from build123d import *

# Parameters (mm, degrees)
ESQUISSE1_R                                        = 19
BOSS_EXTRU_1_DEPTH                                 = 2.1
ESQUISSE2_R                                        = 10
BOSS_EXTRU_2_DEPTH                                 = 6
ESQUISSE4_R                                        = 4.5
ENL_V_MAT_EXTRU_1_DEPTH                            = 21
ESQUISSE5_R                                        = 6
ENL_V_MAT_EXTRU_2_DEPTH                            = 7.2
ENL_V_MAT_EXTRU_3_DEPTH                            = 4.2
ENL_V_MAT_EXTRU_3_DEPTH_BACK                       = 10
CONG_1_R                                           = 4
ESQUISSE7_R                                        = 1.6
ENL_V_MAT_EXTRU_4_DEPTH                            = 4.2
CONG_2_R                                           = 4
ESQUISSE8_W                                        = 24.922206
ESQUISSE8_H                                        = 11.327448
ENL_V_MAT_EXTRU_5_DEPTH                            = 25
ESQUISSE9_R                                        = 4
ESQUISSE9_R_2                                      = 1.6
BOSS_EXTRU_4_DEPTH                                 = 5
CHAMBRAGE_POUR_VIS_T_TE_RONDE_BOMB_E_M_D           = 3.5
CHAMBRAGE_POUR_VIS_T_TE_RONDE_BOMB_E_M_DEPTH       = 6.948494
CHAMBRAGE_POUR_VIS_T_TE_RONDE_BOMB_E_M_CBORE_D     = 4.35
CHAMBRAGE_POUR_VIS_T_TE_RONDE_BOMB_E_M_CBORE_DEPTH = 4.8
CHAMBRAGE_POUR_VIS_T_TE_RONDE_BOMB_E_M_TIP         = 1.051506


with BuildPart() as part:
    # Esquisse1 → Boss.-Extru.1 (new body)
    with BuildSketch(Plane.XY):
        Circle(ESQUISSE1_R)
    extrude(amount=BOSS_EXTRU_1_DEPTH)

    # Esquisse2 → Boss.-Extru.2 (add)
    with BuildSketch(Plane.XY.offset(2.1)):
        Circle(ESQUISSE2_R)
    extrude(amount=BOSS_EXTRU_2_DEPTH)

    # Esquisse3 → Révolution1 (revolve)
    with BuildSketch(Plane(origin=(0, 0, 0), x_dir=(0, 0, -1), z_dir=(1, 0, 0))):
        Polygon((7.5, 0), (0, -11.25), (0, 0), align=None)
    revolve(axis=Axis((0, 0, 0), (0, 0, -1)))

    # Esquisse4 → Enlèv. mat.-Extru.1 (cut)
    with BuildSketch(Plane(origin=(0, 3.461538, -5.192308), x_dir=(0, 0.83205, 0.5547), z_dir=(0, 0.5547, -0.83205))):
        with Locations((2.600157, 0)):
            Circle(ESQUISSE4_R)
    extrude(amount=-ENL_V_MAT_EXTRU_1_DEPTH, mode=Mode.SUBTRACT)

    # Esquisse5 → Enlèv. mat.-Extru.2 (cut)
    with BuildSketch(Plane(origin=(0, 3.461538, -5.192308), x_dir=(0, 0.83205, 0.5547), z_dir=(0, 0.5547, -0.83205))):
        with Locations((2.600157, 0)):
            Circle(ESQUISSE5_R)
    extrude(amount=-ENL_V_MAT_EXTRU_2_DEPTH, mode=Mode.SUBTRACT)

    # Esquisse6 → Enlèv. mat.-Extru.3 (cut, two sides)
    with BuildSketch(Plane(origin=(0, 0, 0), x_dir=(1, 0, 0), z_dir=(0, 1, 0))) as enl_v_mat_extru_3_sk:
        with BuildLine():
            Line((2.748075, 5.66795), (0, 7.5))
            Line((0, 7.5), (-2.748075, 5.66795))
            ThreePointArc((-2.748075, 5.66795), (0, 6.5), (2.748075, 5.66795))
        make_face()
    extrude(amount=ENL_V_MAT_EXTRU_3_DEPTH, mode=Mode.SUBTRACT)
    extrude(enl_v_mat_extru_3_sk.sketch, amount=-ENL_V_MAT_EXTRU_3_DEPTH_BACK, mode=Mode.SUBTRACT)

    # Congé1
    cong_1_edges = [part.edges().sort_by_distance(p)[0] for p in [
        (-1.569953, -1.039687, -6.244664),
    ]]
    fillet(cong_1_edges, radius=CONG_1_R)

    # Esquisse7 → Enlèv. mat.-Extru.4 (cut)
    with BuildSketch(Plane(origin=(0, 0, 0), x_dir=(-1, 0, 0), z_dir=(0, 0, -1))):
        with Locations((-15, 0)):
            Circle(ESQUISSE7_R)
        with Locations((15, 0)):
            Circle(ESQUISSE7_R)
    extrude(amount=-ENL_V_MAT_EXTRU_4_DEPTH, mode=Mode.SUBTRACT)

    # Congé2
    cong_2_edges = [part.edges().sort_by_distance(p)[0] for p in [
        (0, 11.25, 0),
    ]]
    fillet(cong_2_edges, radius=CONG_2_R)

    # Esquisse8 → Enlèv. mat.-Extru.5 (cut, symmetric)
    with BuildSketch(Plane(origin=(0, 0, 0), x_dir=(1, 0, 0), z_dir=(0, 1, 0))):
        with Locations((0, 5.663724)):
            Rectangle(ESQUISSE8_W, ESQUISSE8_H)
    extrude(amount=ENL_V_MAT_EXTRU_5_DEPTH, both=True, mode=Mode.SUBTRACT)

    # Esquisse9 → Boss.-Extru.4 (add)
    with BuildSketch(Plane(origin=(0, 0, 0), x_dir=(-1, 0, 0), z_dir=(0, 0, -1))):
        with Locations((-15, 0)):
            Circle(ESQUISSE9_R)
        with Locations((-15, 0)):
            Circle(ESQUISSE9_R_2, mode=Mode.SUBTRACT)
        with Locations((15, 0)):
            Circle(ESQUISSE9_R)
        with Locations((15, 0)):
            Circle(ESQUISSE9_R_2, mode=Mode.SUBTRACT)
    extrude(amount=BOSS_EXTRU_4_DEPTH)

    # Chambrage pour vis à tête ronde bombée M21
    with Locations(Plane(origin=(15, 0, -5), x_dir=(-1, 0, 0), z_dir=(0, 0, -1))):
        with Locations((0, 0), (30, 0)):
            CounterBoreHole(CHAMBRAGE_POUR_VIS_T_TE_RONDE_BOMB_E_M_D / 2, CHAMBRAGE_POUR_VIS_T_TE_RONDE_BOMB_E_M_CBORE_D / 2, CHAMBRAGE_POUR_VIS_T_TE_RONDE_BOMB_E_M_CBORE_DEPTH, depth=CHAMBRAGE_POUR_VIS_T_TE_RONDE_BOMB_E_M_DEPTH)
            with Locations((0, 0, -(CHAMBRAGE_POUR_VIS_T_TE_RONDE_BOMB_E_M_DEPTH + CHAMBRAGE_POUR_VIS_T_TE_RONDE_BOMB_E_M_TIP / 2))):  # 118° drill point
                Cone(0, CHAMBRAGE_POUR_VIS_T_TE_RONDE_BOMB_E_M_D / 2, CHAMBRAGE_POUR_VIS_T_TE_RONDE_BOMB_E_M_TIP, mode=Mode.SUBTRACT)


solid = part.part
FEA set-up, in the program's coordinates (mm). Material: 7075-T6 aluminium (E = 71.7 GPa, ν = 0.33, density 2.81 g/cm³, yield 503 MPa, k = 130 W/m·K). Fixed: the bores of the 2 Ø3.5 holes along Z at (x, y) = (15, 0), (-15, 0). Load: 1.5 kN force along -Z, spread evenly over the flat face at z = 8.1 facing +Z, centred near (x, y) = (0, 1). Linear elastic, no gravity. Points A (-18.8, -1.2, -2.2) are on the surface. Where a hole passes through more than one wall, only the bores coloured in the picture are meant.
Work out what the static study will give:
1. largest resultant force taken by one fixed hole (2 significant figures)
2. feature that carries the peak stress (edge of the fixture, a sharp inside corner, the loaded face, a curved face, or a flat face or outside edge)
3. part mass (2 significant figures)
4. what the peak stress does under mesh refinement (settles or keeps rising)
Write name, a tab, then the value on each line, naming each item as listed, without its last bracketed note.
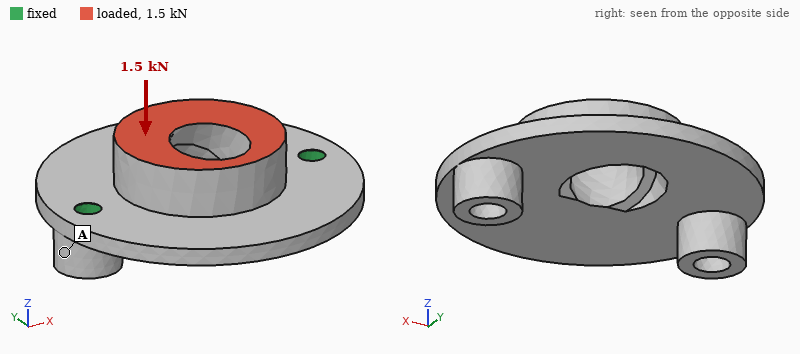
largest resultant force taken by one fixed hole	930 N
feature that carries the peak stress	edge of the fixture
part mass	11 g
what the peak stress does under mesh refinement	keeps rising
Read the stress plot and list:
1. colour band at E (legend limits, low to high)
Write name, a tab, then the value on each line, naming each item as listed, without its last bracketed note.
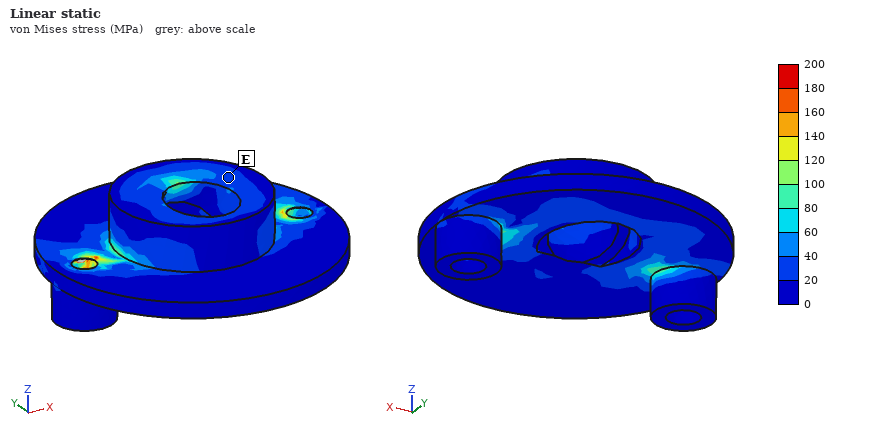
colour band at E	20 to 40 MPa
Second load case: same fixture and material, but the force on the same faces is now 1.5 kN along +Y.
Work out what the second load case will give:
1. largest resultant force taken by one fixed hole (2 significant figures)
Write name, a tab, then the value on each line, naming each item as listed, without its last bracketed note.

largest resultant force taken by one fixed hole	750 N
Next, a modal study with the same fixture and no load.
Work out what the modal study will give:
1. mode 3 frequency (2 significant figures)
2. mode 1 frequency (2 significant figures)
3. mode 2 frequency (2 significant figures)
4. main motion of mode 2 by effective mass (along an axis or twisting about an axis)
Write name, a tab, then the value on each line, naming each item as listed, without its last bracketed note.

mode 3 frequency	18 kHz
mode 1 frequency	5700 Hz
mode 2 frequency	11 kHz
main motion of mode 2 by effective mass	along Z
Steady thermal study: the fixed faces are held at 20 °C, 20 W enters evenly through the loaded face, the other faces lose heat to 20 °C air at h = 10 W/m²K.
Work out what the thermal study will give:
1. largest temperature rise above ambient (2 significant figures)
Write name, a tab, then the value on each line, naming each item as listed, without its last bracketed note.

largest temperature rise above ambient	22 K
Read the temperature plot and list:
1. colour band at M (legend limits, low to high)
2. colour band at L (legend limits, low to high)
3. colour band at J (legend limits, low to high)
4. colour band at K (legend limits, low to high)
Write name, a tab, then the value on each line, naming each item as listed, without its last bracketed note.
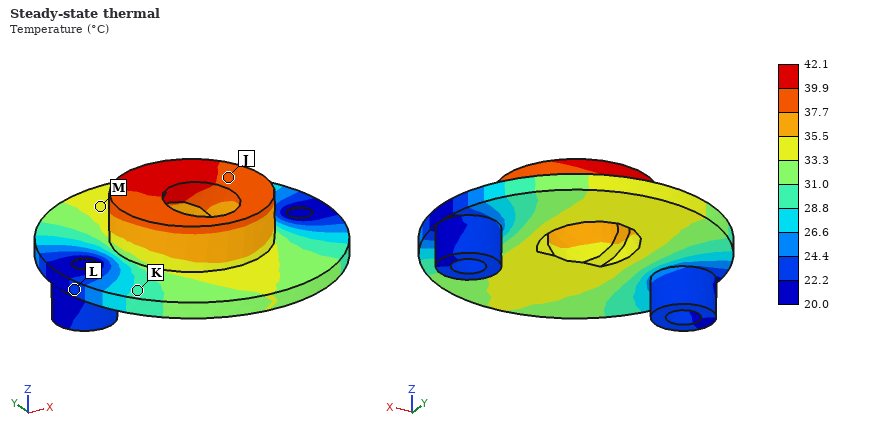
colour band at M	33.3 to 35.5 °C
colour band at L	22.2 to 24.4 °C
colour band at J	37.7 to 39.9 °C
colour band at K	28.8 to 31.0 °C
